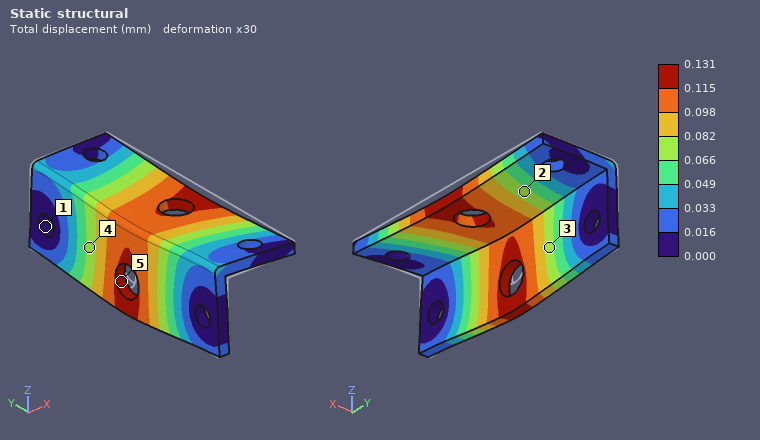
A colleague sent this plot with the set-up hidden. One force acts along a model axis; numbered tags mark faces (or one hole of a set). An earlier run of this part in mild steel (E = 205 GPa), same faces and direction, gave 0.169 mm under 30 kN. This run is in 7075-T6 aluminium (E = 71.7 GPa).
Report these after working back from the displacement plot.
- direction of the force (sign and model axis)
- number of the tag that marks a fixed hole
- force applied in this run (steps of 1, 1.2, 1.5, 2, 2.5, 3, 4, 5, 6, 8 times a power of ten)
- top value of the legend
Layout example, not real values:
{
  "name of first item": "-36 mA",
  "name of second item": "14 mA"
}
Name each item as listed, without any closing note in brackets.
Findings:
{
  "direction of the force": "-Z",
  "number of the tag that marks a fixed hole": "1",
  "force applied in this run": "8 kN",
  "top value of the legend": "0.131 mm"
}
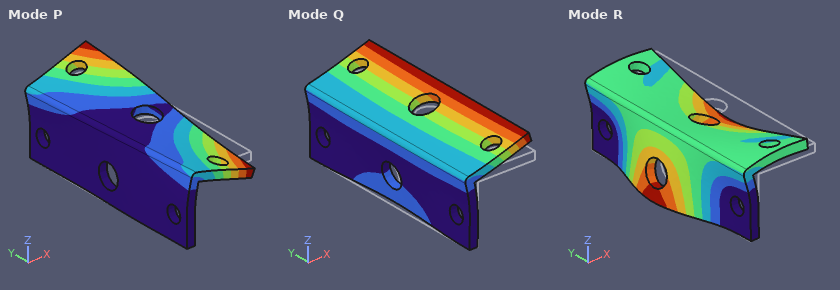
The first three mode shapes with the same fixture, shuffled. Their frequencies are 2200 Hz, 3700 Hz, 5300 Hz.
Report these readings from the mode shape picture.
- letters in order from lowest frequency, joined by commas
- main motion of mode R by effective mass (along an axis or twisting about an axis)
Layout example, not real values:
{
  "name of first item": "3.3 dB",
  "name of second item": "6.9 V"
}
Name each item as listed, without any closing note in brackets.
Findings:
{
  "letters in order from lowest frequency, joined by commas": "Q, P, R",
  "main motion of mode R by effective mass": "along X"
}
